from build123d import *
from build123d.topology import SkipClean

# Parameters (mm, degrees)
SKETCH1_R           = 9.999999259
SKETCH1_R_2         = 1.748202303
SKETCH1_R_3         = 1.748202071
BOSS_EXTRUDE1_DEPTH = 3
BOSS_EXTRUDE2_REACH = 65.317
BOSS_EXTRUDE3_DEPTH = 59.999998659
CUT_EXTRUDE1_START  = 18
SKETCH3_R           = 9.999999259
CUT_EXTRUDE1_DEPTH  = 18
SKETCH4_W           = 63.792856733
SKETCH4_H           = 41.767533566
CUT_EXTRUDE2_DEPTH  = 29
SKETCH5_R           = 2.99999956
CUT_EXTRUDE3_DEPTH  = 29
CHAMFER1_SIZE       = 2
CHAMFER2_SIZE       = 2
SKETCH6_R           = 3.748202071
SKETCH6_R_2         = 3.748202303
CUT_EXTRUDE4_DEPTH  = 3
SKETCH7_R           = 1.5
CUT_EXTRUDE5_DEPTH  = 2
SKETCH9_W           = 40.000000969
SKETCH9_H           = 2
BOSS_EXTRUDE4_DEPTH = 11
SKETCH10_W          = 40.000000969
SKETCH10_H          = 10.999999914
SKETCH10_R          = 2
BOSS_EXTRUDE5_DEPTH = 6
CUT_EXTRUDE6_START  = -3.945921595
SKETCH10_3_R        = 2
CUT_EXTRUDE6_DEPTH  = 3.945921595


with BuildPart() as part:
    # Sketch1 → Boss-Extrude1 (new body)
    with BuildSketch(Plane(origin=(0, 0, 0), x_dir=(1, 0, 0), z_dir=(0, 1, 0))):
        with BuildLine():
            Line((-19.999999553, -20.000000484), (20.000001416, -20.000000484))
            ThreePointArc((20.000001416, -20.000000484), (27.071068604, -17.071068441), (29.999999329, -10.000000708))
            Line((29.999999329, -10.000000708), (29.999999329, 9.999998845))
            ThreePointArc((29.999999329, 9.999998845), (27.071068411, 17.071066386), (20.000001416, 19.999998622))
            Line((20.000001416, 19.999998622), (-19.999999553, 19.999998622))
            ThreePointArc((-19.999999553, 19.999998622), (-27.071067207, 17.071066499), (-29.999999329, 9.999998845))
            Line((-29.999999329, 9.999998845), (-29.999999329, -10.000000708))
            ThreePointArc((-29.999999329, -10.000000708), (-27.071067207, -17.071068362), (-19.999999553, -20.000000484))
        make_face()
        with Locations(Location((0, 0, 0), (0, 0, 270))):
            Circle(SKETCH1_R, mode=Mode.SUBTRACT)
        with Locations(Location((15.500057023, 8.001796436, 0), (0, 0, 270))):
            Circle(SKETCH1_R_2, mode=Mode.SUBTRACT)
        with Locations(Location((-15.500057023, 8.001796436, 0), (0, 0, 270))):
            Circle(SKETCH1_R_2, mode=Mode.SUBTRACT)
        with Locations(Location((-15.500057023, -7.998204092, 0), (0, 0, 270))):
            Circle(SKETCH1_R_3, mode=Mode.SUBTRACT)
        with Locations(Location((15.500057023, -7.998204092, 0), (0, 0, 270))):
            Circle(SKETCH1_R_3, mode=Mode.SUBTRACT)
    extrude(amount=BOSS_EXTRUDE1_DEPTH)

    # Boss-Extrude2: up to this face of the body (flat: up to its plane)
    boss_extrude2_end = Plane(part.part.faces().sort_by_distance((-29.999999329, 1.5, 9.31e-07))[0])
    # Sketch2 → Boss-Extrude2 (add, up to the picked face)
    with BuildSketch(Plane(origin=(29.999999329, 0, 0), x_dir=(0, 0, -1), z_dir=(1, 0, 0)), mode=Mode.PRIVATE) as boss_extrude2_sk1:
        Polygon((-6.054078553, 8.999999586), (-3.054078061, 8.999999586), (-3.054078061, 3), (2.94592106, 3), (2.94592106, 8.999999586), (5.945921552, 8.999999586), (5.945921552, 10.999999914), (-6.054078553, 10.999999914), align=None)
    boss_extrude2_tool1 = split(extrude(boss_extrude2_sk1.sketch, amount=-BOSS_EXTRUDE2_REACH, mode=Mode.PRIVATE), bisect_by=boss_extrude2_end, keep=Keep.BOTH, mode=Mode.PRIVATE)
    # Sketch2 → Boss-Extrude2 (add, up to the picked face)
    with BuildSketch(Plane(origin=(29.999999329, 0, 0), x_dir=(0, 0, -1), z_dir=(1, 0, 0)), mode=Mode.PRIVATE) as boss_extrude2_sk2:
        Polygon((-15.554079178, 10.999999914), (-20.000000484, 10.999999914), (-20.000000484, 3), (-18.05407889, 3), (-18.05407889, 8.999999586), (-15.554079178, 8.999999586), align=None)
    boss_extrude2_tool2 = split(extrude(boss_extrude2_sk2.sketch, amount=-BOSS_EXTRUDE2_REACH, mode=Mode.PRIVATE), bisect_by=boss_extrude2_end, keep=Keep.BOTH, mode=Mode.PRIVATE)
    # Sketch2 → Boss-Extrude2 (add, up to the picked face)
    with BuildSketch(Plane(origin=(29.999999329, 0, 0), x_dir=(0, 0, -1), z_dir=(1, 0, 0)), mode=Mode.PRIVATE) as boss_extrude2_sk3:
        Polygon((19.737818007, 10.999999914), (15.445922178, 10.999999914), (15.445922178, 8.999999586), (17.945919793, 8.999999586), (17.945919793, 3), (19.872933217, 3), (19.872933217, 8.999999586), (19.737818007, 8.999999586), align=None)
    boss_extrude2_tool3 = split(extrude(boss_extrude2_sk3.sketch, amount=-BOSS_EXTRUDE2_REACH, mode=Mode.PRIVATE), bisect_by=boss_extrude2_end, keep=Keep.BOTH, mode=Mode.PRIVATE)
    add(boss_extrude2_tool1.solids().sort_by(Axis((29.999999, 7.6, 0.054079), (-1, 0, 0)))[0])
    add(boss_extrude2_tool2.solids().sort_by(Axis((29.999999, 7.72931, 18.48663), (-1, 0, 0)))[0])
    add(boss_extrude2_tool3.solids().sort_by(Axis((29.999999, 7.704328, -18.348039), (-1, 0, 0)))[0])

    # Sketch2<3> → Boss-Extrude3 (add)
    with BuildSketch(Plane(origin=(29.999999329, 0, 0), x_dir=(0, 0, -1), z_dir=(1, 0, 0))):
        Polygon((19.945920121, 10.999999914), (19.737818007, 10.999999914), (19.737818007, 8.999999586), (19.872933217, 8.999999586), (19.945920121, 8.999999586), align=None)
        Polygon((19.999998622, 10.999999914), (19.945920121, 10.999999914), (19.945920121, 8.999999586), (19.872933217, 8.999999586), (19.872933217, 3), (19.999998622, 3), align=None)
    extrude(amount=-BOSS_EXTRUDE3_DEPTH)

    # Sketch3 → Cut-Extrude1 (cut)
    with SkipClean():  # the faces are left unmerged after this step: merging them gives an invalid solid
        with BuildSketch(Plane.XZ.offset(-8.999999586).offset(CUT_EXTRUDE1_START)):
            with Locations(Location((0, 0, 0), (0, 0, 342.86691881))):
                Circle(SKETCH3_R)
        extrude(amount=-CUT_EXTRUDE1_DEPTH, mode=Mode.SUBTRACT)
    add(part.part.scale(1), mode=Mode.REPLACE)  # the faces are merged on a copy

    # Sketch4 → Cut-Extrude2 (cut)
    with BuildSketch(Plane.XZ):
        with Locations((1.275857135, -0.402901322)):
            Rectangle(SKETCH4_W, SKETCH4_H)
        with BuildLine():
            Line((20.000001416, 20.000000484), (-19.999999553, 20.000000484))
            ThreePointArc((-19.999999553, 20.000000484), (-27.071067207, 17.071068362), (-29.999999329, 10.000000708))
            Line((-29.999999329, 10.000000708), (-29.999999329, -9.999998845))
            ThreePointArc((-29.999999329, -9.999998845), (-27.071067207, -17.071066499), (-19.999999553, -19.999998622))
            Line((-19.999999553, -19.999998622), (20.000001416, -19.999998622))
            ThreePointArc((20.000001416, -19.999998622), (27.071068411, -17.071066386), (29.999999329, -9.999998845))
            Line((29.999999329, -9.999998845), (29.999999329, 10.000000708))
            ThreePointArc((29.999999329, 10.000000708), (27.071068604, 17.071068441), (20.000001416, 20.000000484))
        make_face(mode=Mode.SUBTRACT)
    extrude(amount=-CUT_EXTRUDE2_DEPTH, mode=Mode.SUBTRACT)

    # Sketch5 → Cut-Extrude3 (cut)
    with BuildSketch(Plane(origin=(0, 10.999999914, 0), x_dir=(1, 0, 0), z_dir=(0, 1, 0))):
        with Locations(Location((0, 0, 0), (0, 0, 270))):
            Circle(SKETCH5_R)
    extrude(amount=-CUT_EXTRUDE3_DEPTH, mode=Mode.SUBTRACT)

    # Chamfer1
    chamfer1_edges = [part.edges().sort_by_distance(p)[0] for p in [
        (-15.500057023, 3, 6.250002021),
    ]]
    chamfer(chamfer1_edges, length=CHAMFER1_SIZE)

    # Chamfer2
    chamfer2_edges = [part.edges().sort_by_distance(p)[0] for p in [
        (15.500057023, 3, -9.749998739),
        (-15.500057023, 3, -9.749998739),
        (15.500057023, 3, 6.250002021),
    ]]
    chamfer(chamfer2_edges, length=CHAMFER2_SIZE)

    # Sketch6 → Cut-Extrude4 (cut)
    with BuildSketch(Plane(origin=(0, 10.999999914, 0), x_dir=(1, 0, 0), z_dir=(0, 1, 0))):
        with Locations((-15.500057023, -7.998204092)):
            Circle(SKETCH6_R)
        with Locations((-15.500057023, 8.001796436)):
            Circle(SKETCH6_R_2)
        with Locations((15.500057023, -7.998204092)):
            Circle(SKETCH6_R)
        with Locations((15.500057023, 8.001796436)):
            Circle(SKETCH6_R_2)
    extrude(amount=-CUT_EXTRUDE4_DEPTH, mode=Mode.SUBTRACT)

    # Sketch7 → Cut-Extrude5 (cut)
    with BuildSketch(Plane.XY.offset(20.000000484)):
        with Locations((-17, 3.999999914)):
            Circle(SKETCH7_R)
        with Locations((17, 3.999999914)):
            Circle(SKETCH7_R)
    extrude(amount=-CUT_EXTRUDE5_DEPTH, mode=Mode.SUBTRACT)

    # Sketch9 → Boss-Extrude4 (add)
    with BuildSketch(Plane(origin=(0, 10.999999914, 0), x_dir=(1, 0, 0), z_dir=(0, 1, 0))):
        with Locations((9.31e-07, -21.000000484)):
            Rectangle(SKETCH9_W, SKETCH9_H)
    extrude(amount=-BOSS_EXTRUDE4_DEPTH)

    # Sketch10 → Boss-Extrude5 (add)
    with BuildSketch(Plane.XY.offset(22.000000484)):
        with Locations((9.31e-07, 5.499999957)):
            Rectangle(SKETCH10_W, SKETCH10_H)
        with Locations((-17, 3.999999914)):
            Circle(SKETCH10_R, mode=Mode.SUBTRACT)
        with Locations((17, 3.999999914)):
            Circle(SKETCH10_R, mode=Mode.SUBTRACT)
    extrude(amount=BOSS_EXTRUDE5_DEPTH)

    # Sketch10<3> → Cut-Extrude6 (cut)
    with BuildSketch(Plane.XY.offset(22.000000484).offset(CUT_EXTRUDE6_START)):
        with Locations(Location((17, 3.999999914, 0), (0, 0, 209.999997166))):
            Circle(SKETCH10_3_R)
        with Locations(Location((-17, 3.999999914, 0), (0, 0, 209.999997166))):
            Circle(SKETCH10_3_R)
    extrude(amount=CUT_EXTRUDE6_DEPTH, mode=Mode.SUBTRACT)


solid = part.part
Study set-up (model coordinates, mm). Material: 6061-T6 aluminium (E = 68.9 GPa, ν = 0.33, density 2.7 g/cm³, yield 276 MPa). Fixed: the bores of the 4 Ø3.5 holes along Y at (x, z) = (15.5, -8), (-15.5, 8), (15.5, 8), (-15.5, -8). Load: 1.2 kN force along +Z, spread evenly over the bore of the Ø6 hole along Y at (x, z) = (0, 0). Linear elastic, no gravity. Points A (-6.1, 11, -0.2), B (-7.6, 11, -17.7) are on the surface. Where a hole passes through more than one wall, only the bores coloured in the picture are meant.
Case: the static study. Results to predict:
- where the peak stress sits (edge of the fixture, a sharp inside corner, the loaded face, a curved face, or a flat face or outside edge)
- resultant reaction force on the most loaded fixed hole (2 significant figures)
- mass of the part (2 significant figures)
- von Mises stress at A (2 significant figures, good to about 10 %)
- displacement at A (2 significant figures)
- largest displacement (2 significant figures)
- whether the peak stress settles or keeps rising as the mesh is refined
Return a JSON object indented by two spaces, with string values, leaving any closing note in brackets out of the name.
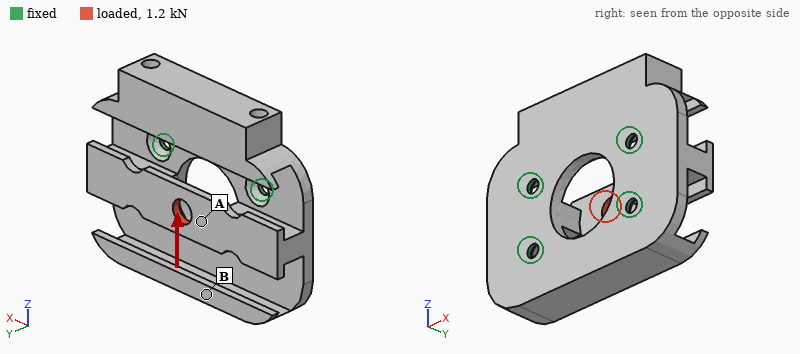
{
  "where the peak stress sits": "edge of the fixture",
  "resultant reaction force on the most loaded fixed hole": "520 N",
  "mass of the part": "38 g",
  "von Mises stress at A": "66 MPa",
  "displacement at A": "41 µm",
  "largest displacement": "53 µm",
  "whether the peak stress settles or keeps rising as the mesh is refined": "keeps rising"
}
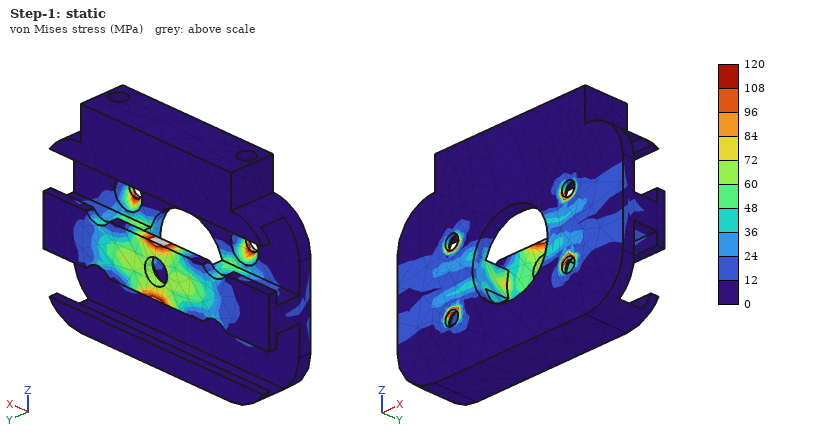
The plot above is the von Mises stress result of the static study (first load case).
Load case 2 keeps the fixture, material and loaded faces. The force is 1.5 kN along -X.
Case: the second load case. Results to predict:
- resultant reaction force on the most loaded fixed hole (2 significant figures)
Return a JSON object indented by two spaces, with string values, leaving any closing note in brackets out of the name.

{
  "resultant reaction force on the most loaded fixed hole": "450 N"
}
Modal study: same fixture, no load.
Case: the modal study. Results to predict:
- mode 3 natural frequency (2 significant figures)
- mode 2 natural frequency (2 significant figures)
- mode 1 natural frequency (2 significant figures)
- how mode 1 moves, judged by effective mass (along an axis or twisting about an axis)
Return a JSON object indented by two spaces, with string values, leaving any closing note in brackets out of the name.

{
  "mode 3 natural frequency": "6700 Hz",
  "mode 2 natural frequency": "5700 Hz",
  "mode 1 natural frequency": "2500 Hz",
  "how mode 1 moves, judged by effective mass": "along Y"
}
